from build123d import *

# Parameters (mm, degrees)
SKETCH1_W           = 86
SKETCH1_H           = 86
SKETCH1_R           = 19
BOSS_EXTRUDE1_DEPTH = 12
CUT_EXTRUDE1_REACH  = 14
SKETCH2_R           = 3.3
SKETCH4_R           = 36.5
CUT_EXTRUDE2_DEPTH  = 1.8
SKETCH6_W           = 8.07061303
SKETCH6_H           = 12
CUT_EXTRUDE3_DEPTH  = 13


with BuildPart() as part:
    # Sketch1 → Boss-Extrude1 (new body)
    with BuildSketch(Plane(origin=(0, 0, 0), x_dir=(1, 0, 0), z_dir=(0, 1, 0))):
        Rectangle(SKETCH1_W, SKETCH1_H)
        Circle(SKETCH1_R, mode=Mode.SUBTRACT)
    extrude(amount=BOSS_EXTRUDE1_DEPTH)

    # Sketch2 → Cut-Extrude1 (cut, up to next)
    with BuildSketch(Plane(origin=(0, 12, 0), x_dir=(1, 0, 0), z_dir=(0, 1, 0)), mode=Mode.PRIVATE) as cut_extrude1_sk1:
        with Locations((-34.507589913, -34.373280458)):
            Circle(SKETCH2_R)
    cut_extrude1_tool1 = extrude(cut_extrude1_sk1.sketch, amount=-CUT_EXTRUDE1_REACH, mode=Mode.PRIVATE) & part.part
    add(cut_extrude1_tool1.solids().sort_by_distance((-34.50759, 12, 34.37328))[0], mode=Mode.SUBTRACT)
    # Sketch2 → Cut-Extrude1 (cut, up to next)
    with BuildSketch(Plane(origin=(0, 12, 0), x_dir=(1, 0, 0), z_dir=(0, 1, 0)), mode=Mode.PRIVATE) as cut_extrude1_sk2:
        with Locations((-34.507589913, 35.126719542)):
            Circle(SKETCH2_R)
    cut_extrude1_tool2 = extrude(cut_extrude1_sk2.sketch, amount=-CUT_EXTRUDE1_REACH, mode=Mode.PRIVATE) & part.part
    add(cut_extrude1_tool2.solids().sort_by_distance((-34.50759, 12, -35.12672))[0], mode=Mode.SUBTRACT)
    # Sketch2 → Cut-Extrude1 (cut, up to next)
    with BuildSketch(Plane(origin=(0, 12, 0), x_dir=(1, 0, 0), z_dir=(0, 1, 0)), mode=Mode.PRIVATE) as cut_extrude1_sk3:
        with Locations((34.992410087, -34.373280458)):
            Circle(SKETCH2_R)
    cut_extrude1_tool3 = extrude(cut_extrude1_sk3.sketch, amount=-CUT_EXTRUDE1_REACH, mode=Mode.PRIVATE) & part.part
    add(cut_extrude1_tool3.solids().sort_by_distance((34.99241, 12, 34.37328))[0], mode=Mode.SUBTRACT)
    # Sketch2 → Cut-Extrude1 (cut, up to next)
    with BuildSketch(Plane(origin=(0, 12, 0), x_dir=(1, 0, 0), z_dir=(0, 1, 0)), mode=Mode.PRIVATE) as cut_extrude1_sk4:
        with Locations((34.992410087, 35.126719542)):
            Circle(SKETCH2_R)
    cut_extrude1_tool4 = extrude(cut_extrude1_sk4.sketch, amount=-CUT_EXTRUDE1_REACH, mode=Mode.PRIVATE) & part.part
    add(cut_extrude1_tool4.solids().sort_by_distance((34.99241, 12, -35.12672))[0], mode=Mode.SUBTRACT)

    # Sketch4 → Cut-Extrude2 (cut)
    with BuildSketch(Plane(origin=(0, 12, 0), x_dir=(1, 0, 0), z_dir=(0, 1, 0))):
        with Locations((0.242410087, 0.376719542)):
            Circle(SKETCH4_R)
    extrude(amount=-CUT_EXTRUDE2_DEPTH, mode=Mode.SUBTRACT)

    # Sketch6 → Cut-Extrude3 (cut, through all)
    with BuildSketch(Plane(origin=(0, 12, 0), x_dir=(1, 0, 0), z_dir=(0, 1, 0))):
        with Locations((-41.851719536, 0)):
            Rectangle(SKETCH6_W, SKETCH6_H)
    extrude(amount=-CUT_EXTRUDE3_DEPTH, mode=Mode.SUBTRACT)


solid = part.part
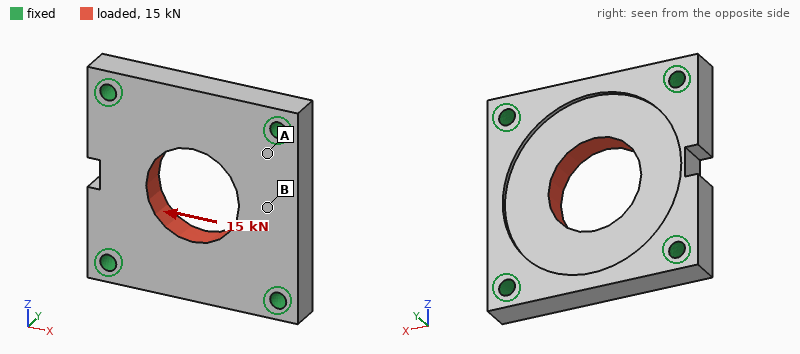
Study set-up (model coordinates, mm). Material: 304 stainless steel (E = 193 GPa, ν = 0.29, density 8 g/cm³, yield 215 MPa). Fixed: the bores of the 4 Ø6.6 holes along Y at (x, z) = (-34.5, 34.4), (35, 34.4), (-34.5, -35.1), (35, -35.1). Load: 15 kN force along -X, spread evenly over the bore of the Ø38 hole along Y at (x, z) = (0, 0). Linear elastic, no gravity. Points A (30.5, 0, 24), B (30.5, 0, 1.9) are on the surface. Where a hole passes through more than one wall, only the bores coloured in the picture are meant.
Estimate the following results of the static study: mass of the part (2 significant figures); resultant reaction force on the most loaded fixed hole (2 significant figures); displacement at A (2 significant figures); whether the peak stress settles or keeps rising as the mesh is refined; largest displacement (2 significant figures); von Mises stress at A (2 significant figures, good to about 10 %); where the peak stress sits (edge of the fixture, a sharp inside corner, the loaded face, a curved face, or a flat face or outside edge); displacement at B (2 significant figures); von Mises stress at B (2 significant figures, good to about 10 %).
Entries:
540 g
4.2 kN
1.7 µm
keeps rising
5.4 µm
18 MPa
edge of the fixture
4.3 µm
6.8 MPa
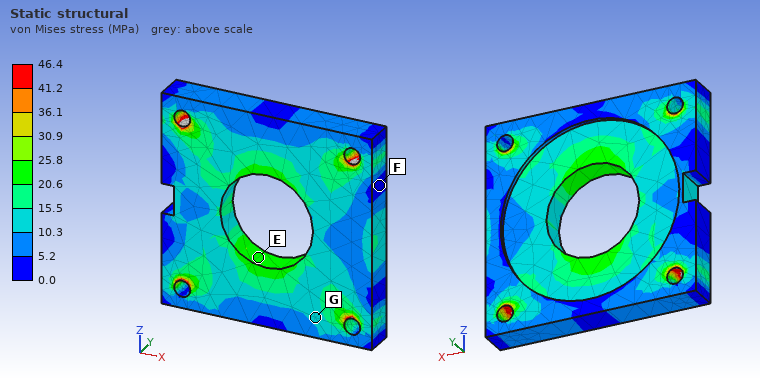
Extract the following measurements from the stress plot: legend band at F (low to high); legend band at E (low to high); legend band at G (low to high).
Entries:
0.0 to 5.2 MPa
20.6 to 25.8 MPa
10.3 to 15.5 MPa
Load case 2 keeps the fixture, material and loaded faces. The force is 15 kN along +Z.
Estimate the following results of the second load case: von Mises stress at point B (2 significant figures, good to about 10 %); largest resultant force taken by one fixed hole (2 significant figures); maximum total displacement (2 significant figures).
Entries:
13 MPa
4.1 kN
5.0 µm
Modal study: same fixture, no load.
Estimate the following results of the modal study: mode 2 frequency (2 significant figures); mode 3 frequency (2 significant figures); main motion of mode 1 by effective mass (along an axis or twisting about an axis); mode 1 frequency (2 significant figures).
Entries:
11 kHz
11 kHz
along Y
8500 Hz
